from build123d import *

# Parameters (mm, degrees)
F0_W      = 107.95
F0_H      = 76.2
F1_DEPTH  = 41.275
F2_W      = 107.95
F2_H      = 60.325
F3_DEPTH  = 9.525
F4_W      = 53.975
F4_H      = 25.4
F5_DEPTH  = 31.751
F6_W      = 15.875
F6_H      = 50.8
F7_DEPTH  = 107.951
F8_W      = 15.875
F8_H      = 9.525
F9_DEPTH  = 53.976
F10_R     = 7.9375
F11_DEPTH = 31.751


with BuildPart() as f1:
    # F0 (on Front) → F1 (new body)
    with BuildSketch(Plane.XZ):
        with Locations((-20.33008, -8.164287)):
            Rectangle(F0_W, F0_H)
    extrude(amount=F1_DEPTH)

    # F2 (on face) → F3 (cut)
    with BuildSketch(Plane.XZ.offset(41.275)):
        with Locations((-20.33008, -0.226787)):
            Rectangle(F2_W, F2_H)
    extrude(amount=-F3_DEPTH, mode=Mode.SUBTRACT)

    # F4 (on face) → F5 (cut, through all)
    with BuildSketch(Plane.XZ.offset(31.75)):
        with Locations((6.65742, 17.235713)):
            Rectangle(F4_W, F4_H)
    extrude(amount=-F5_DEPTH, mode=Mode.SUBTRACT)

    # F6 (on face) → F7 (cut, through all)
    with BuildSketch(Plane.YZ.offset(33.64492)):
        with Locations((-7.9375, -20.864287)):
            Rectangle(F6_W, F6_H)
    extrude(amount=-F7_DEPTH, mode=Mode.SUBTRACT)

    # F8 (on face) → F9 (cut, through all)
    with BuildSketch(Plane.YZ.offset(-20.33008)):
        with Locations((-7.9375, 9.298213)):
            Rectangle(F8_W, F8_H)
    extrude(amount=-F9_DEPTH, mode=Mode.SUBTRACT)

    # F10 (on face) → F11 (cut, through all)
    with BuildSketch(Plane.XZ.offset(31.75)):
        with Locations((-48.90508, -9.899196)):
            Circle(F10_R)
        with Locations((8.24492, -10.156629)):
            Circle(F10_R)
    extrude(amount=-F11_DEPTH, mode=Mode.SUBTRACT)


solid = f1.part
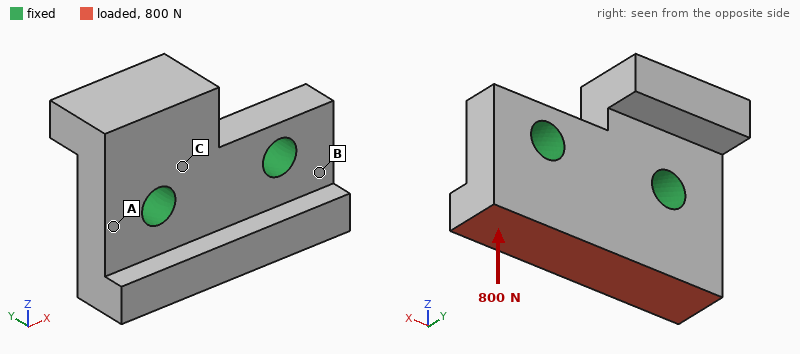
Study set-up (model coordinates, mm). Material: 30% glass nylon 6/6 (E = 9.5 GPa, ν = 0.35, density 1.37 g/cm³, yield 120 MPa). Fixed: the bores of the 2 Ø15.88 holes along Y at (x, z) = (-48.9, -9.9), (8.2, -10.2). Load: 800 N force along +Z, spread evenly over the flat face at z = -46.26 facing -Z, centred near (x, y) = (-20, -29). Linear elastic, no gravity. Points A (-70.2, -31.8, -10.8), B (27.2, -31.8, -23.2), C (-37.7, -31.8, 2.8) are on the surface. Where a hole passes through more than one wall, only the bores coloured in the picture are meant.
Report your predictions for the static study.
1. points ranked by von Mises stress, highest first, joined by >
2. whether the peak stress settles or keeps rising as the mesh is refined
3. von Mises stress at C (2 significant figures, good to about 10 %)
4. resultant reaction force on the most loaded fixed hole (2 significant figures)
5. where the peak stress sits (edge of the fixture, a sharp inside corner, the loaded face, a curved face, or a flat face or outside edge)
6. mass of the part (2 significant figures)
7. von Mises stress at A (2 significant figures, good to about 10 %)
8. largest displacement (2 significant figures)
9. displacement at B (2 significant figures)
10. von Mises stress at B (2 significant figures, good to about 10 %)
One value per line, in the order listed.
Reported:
B > A > C
keeps rising
0.24 MPa
410 N
edge of the fixture
180 g
0.58 MPa
8.9 µm
2.5 µm
0.94 MPa
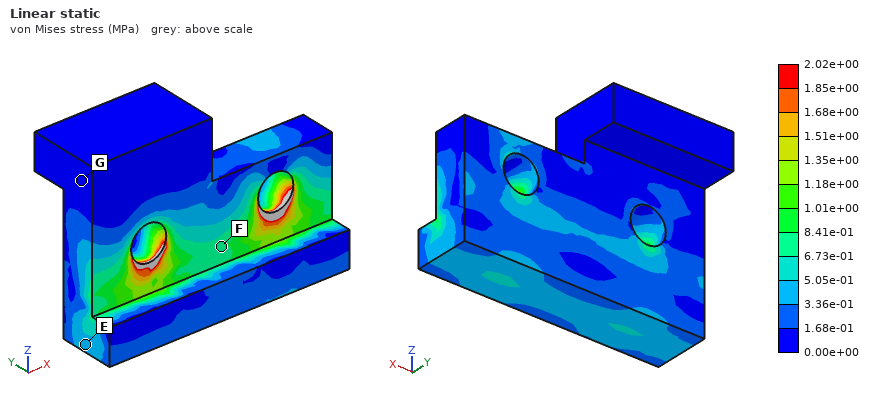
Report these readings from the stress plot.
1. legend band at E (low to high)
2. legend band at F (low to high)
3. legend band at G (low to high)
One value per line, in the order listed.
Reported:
3.36e-01 to 5.05e-01 MPa
6.73e-01 to 8.41e-01 MPa
0.00e+00 to 1.68e-01 MPa
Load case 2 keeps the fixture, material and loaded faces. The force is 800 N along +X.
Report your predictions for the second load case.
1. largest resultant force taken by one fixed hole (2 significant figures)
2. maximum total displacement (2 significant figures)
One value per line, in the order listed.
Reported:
560 N
10 µm
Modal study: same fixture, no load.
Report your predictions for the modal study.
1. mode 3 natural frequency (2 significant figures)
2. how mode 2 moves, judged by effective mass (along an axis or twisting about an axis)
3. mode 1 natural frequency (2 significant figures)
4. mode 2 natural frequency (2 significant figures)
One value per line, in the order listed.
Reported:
4100 Hz
along Y
2900 Hz
3900 Hz
